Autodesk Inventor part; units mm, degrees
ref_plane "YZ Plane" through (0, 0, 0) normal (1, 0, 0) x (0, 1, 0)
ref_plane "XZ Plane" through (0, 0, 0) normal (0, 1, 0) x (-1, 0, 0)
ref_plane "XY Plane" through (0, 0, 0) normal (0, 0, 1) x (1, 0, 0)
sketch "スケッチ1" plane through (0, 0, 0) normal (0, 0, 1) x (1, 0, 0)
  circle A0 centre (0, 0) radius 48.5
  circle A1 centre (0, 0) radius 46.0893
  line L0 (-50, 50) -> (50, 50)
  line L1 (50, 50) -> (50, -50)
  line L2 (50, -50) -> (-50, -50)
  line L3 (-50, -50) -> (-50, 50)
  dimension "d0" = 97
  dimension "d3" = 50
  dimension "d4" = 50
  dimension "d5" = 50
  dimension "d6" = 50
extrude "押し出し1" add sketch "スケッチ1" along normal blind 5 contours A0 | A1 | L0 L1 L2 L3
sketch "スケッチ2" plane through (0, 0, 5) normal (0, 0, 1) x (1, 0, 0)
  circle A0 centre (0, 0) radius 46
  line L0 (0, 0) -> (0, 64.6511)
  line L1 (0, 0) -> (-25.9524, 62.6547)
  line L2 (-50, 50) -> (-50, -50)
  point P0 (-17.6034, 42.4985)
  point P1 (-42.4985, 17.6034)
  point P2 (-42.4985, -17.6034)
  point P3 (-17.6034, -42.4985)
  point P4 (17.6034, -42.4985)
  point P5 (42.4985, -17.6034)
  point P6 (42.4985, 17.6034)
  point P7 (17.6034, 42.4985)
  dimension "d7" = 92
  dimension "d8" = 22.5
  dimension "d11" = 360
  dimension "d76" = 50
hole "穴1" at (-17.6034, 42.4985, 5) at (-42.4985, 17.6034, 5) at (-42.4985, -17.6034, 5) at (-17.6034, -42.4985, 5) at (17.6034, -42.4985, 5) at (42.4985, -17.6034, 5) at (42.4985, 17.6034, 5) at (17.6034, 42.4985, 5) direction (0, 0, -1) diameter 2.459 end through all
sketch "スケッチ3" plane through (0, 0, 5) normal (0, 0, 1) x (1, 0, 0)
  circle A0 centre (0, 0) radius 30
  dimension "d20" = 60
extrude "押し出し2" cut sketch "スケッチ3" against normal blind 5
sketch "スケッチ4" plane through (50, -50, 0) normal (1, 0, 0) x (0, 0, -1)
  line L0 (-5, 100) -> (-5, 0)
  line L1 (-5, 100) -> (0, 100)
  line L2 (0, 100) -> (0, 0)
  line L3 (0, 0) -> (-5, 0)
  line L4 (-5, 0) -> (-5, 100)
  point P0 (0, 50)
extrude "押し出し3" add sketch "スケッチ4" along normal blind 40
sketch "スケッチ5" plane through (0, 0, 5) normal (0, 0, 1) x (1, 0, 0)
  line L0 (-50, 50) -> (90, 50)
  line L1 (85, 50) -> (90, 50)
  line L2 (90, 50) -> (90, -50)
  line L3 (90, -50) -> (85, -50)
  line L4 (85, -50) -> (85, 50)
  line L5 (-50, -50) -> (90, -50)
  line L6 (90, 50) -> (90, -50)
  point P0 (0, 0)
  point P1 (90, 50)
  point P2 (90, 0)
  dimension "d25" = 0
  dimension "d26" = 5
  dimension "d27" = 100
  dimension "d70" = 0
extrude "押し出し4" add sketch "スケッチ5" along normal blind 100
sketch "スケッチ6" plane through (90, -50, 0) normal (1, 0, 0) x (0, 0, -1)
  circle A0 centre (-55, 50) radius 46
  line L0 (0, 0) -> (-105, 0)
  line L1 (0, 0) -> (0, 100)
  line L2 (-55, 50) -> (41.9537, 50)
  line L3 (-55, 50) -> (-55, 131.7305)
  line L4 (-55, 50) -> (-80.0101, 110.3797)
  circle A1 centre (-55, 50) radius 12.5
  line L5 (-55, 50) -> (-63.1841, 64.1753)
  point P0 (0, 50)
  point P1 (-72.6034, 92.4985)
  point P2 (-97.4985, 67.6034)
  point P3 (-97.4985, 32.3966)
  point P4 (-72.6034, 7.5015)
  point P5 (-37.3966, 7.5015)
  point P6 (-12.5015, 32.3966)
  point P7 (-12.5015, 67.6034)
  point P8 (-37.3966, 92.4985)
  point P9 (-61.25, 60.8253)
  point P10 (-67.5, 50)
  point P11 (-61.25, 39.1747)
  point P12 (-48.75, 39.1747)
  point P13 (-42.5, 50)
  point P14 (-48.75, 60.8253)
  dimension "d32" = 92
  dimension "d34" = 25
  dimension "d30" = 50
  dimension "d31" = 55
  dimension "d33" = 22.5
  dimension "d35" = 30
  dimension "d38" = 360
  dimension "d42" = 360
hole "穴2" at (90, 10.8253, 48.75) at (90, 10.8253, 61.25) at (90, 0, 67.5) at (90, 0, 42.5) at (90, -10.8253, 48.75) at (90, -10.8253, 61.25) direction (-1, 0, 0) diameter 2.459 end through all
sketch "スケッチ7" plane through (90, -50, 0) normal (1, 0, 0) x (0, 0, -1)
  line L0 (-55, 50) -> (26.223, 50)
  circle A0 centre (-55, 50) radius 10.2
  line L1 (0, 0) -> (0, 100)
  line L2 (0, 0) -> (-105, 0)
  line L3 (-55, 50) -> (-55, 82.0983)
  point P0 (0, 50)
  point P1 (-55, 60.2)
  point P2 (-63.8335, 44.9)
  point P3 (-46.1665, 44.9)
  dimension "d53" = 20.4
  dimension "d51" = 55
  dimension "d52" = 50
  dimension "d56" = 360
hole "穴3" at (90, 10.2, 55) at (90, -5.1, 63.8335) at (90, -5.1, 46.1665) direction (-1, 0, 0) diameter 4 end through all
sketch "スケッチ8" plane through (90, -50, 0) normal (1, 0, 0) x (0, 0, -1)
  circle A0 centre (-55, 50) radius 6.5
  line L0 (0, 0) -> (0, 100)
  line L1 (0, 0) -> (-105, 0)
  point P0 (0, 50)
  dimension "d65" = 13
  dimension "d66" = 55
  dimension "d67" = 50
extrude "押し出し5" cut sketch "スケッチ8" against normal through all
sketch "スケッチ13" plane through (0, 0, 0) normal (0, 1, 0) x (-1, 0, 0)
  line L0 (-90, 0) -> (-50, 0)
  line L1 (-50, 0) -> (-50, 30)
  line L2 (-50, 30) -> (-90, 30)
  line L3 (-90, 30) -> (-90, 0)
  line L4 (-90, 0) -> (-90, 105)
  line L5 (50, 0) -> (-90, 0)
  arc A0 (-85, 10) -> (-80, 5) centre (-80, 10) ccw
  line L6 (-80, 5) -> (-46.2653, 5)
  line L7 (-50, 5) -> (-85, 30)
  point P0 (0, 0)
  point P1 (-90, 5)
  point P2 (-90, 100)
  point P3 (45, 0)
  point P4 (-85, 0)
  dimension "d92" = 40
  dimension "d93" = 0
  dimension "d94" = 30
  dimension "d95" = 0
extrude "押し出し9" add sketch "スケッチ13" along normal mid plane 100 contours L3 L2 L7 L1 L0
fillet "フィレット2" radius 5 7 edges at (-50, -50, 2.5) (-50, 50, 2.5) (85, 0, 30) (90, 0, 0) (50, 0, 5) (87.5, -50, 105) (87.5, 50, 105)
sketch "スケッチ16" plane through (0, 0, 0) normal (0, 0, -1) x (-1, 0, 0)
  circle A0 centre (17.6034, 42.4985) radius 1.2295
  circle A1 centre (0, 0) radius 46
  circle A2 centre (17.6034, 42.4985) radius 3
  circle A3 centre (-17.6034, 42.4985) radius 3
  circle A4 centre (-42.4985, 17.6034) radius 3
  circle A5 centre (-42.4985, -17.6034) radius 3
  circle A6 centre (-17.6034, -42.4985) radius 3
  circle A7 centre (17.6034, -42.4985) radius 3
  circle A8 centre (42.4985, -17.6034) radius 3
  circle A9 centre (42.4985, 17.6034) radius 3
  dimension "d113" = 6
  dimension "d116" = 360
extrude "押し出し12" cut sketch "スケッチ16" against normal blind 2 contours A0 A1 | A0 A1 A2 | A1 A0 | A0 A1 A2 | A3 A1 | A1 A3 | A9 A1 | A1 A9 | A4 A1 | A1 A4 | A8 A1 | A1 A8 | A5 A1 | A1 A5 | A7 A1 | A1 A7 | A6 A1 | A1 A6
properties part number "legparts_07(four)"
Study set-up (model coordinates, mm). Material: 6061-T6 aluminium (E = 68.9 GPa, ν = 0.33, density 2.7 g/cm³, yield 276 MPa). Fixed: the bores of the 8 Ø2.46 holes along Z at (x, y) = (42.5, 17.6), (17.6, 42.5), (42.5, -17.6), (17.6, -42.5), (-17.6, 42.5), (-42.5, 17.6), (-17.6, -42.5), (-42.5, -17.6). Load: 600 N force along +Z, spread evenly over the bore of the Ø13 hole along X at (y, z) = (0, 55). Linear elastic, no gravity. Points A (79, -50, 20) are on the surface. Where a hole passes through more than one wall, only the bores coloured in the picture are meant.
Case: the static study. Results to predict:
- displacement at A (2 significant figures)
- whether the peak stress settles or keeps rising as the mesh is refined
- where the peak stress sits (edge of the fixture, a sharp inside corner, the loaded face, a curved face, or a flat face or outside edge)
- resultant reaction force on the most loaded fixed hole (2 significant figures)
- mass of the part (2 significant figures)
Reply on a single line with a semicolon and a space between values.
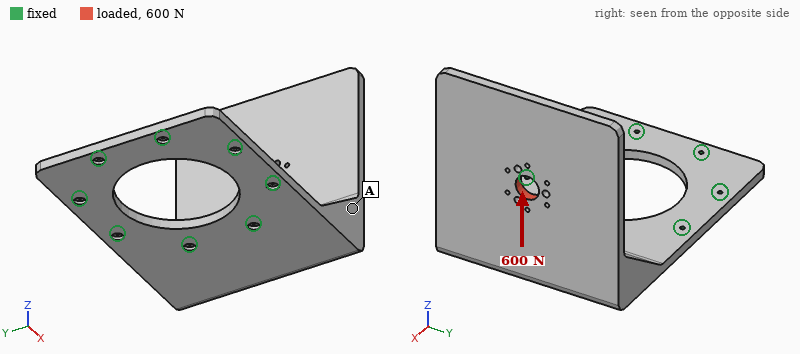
0.28 mm; keeps rising; edge of the fixture; 780 N; 400 g
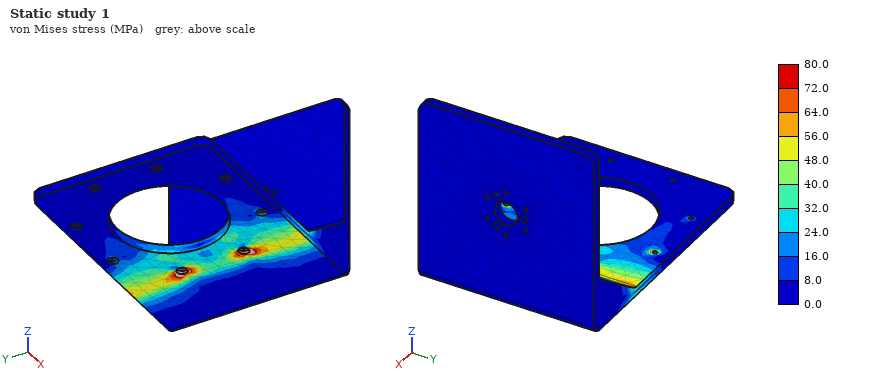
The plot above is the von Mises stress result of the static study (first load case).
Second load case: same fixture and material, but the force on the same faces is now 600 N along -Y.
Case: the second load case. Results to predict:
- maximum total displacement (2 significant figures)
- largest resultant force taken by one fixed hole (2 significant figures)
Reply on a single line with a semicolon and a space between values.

0.15 mm; 750 N
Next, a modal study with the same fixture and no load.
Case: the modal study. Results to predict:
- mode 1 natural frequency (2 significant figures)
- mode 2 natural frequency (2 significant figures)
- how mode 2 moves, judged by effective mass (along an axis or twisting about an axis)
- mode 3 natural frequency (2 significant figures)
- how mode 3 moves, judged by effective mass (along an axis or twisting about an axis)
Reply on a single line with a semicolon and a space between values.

300 Hz; 910 Hz; along Y; 960 Hz; along Z
